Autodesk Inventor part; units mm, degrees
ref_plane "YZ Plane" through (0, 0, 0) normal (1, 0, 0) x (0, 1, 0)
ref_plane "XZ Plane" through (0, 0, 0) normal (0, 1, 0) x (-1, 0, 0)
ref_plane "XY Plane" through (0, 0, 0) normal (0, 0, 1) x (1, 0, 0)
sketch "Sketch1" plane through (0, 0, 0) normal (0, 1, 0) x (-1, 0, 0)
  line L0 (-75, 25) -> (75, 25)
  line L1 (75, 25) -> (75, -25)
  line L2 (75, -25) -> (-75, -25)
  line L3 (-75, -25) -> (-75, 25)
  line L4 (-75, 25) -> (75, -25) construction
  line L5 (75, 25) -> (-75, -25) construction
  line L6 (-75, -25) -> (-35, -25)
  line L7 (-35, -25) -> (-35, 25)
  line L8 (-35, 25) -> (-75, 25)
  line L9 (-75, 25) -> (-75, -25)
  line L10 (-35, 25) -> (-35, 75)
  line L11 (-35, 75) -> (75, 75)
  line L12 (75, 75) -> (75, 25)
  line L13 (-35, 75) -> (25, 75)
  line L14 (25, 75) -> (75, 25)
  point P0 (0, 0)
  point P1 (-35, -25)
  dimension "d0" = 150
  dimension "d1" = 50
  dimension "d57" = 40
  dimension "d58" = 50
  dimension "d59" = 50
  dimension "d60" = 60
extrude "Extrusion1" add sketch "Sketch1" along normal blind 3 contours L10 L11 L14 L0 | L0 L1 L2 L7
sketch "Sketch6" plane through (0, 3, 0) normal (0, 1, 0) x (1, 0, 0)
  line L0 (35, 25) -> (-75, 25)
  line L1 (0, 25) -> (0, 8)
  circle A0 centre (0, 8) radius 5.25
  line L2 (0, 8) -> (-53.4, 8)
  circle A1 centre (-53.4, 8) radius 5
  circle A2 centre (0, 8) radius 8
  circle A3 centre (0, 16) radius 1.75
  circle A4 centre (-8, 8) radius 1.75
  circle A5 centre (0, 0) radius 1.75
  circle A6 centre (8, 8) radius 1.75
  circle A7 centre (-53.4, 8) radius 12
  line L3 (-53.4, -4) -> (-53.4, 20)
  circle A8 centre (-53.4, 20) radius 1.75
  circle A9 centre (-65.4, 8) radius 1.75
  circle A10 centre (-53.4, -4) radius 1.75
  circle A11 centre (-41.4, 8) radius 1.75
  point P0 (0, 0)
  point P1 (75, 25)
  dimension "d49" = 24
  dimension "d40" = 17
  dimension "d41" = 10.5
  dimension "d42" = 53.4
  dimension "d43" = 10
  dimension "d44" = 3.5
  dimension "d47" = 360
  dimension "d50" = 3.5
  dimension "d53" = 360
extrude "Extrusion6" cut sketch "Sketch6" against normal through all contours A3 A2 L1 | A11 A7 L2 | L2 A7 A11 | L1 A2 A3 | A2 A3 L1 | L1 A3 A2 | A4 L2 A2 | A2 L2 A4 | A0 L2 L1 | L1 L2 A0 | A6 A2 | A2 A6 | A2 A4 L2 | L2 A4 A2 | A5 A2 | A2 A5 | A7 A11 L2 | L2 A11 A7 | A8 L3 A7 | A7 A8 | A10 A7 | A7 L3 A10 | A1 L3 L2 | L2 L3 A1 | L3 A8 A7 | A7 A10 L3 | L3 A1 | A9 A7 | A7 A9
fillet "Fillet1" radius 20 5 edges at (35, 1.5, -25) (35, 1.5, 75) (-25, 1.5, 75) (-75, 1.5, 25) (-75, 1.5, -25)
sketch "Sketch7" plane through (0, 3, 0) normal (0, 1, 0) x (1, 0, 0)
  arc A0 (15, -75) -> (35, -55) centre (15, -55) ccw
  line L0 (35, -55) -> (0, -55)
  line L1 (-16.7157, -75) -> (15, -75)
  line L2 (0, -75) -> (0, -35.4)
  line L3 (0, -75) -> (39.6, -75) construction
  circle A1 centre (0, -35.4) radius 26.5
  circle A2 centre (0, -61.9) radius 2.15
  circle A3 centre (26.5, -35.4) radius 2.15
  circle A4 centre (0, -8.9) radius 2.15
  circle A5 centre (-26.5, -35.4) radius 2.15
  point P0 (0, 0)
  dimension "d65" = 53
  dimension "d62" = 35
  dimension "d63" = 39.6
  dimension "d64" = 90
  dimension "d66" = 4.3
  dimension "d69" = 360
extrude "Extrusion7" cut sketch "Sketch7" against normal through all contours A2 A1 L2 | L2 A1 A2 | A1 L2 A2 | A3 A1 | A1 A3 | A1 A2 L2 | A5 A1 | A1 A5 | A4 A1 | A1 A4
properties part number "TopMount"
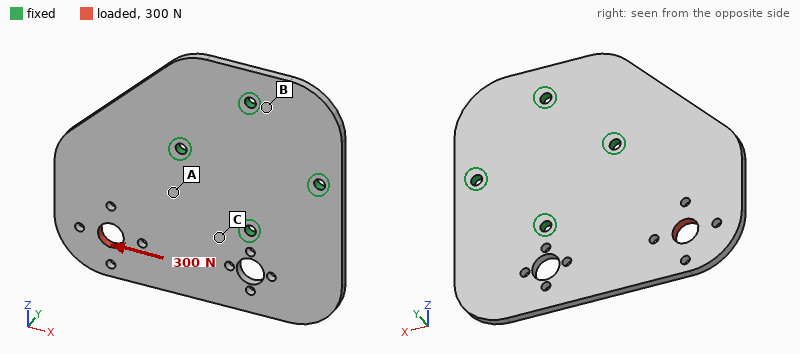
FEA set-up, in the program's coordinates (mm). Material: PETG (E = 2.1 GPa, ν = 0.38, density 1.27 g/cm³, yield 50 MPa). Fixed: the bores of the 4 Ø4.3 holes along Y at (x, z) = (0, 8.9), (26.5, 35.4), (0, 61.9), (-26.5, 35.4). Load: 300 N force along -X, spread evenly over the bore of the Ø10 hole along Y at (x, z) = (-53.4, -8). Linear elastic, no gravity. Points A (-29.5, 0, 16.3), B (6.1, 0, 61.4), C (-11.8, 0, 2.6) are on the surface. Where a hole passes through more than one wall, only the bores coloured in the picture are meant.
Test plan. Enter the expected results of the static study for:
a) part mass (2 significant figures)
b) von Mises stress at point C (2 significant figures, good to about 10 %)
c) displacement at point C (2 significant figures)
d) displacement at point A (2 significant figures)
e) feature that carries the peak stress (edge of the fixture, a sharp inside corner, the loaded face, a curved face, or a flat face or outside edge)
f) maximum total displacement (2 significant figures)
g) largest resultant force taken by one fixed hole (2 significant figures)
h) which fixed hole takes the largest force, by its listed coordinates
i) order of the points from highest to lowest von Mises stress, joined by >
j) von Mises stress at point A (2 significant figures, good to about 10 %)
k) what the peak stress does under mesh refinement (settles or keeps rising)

35 g
3.9 MPa
0.037 mm
0.036 mm
edge of the fixture
0.17 mm
270 N
(0, 8.9)
C > A > B
2.1 MPa
keeps rising
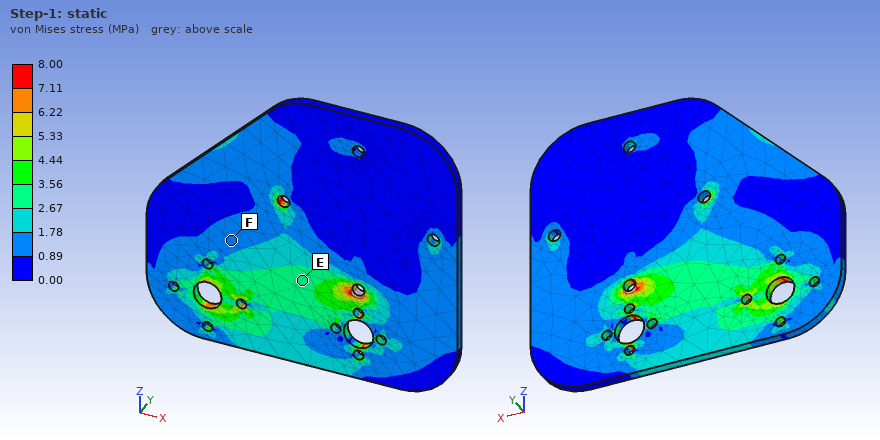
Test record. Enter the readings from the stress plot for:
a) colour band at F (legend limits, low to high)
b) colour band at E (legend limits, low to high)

0.89 to 1.78 MPa
2.67 to 3.56 MPa
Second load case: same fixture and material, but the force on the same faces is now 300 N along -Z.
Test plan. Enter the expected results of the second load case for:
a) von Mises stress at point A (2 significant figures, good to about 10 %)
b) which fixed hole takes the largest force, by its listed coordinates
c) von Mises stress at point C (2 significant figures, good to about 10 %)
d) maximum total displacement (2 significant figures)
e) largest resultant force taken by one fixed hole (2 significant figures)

3.2 MPa
(-26.5, 35.4)
1.8 MPa
0.19 mm
290 N
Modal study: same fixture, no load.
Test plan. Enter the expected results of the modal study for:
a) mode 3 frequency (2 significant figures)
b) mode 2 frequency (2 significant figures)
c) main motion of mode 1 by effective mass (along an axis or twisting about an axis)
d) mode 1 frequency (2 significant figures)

490 Hz
410 Hz
along Y
180 Hz
